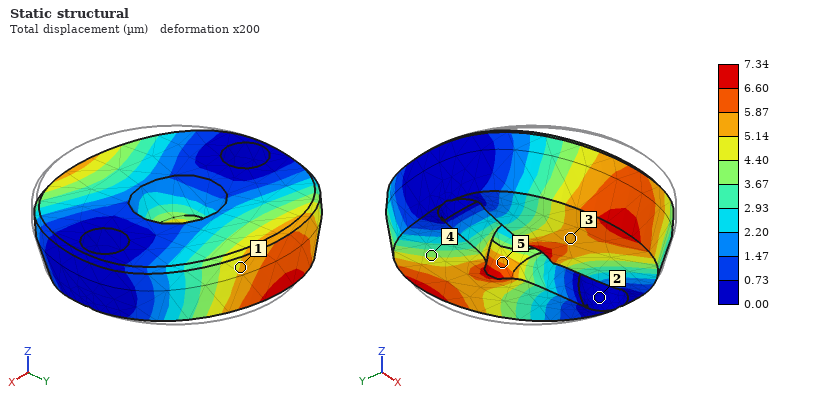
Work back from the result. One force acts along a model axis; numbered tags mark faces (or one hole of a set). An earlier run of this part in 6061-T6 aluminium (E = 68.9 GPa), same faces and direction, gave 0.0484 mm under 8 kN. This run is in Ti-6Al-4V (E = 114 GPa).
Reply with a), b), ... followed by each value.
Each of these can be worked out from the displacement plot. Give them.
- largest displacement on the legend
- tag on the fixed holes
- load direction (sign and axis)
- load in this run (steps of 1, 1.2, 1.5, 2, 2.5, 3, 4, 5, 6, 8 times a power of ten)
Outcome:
a) 7.34 µm
b) 2
c) +Y
d) 2 kN
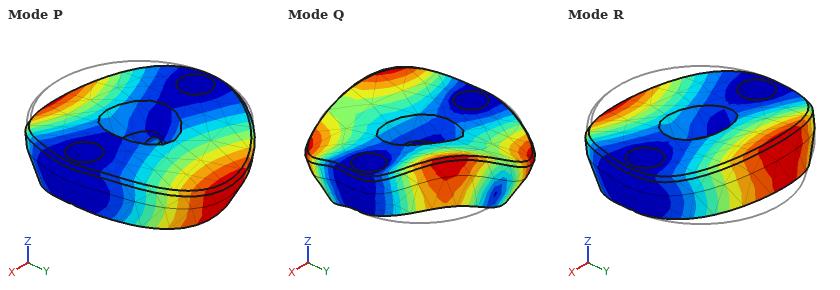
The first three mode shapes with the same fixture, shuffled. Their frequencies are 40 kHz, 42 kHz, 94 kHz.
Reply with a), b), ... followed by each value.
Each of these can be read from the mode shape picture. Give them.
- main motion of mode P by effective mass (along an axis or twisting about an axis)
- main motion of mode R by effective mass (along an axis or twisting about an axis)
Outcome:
a) along Z
b) twisting about X
